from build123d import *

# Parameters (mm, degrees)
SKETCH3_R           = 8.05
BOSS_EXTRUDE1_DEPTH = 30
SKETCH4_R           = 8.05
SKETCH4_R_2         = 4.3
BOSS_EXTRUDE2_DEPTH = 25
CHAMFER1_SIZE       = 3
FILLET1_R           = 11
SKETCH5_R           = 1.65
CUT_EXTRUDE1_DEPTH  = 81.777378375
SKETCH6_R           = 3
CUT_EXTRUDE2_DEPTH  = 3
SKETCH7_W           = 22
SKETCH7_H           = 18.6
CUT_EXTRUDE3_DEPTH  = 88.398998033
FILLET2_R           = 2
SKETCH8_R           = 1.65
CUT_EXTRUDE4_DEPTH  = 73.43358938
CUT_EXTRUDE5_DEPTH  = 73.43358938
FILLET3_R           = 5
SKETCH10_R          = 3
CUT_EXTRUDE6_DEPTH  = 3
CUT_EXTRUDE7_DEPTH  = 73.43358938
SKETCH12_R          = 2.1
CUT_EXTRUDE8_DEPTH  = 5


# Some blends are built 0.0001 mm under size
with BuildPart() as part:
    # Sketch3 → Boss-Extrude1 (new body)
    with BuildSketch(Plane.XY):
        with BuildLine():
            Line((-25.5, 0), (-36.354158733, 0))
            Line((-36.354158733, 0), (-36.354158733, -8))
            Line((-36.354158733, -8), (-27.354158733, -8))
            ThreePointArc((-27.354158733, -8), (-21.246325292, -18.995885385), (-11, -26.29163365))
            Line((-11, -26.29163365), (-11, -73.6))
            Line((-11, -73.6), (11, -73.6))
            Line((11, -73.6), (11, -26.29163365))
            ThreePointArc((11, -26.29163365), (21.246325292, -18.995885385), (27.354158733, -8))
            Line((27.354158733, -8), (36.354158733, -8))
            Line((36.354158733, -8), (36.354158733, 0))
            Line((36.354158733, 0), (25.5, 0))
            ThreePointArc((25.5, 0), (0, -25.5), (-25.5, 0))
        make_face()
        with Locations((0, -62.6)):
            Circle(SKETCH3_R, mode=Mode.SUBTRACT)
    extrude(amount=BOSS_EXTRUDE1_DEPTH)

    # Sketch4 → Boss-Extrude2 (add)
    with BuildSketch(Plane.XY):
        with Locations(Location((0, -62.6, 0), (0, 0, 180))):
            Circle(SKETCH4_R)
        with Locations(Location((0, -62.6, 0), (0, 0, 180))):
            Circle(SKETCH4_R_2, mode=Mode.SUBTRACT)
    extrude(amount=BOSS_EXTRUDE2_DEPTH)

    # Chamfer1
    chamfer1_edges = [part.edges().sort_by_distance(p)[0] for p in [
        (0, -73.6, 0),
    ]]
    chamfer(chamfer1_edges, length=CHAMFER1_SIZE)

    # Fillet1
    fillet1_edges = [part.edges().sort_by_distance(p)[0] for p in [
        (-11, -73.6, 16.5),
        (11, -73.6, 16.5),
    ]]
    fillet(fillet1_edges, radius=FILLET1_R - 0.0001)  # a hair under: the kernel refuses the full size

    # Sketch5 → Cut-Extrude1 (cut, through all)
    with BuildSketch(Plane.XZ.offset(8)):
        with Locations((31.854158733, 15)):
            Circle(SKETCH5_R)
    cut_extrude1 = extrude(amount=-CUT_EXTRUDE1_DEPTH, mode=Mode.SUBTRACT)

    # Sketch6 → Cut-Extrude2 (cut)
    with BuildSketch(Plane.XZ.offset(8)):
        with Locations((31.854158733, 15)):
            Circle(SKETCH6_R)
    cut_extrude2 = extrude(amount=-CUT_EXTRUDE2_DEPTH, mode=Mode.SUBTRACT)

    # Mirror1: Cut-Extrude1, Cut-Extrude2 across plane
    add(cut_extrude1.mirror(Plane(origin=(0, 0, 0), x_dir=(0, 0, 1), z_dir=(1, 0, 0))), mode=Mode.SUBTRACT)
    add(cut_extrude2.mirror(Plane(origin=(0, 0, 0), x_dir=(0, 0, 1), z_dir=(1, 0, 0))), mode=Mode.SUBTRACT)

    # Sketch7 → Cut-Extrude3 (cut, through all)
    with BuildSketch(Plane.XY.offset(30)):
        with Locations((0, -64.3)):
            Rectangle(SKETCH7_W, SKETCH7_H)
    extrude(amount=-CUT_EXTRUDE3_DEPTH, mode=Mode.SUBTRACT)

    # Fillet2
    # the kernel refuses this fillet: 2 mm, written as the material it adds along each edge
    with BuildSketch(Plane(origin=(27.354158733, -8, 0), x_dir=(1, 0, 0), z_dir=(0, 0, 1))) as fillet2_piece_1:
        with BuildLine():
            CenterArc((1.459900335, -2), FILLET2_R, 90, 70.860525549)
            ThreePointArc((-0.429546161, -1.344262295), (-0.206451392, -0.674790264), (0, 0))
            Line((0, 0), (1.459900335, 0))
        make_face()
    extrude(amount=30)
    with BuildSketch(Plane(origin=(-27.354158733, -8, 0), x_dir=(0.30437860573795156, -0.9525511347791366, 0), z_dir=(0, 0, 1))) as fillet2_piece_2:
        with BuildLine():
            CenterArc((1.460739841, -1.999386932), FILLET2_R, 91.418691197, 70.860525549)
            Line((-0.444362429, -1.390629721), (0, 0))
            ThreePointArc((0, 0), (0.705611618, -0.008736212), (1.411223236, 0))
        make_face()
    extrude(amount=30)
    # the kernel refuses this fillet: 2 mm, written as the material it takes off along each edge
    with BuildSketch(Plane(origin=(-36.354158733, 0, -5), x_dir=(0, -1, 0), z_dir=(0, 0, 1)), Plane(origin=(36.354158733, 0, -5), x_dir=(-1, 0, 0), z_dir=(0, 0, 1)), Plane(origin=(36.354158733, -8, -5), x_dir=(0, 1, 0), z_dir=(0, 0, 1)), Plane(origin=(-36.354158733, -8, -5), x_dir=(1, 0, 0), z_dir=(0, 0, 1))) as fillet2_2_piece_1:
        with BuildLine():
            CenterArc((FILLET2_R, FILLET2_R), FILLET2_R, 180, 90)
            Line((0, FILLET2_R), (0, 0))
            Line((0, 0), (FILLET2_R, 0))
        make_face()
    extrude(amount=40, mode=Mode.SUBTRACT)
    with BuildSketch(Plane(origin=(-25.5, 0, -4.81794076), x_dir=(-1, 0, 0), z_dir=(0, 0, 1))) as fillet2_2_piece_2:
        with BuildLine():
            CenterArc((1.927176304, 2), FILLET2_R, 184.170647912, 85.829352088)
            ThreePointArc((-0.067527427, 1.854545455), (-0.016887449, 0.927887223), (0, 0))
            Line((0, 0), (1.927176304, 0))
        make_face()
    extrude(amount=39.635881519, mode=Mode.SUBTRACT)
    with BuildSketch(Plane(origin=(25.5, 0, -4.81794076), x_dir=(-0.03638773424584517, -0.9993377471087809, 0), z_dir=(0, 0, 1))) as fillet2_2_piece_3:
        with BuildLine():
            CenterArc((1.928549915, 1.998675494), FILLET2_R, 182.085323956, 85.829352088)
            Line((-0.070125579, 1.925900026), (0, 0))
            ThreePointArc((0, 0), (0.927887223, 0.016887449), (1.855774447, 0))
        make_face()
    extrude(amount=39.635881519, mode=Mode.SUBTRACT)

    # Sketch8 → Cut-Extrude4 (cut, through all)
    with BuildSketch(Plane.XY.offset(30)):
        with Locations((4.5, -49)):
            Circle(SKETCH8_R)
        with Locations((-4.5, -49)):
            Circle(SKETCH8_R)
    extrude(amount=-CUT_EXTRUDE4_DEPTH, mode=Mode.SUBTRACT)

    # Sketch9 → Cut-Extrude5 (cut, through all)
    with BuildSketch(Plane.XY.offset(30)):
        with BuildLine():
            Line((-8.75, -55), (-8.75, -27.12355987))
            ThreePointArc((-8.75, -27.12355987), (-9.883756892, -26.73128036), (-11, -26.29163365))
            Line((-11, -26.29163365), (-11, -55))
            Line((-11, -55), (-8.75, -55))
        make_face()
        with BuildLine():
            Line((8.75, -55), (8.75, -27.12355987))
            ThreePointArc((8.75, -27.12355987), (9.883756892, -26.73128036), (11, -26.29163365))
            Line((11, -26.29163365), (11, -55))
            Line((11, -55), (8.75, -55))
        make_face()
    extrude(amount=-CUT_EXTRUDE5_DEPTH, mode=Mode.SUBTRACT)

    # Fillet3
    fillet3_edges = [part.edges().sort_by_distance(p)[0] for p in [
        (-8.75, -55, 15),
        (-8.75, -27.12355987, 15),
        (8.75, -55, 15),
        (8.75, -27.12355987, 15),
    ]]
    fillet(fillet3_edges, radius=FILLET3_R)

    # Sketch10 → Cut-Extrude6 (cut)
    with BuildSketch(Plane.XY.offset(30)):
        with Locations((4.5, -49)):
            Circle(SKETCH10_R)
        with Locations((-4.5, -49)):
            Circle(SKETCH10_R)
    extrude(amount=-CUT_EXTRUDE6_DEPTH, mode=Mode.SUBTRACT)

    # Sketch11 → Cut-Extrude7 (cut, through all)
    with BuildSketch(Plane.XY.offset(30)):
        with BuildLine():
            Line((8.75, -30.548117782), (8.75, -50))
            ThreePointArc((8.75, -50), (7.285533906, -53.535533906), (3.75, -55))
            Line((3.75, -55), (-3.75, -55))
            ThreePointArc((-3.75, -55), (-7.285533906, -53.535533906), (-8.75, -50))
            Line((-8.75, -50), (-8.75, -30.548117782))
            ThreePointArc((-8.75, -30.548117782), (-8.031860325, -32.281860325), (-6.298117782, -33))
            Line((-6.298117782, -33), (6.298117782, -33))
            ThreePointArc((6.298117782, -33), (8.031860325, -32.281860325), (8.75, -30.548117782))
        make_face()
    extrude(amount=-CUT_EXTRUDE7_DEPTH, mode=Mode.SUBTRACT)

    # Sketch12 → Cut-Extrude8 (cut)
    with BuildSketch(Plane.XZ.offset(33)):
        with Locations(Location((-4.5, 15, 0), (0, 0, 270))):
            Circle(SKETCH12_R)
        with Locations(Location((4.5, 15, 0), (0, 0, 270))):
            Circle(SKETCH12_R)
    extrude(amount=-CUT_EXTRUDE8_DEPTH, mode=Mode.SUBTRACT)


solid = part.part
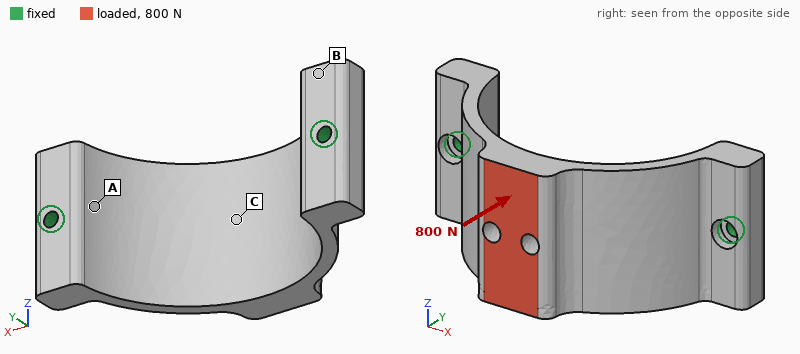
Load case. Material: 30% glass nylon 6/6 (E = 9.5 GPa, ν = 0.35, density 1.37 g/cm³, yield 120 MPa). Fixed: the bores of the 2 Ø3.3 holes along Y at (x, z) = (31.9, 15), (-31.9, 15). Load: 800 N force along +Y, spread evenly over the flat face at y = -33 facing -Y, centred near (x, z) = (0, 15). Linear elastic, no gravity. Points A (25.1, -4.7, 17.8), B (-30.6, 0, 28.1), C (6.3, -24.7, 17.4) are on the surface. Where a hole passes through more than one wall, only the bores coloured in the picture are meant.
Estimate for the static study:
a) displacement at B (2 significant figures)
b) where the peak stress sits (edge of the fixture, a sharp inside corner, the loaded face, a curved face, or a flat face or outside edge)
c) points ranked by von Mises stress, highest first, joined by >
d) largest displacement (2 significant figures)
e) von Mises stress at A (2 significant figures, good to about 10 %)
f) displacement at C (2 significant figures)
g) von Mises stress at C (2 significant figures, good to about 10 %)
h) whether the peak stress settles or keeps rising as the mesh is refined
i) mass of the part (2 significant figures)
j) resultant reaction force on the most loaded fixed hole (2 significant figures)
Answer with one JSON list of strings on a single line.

["14 µm", "edge of the fixture", "C > A > B", "83 µm", "5.1 MPa", "73 µm", "7.1 MPa", "keeps rising", "19 g", "530 N"]
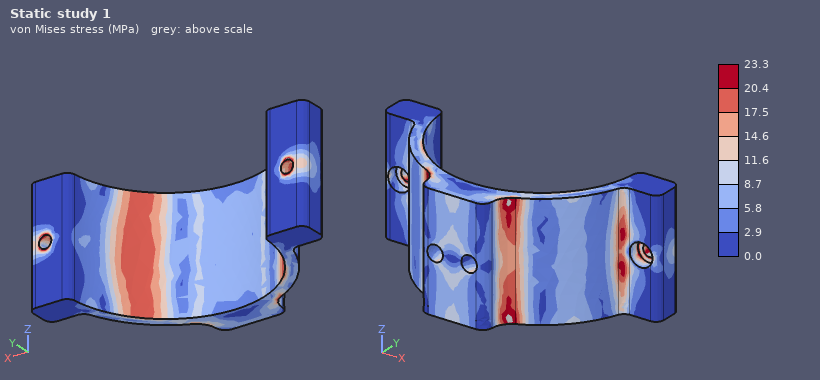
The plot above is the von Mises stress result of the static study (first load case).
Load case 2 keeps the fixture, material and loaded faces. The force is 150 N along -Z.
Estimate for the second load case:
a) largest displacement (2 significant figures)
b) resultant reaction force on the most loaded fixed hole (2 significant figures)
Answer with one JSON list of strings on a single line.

["0.24 mm", "75 N"]
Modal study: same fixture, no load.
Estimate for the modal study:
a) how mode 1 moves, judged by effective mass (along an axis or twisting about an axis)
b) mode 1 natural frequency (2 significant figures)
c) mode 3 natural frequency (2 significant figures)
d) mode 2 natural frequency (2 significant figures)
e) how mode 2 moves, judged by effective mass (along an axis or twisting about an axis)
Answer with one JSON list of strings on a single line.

["along Z", "1600 Hz", "5100 Hz", "2700 Hz", "along X"]
